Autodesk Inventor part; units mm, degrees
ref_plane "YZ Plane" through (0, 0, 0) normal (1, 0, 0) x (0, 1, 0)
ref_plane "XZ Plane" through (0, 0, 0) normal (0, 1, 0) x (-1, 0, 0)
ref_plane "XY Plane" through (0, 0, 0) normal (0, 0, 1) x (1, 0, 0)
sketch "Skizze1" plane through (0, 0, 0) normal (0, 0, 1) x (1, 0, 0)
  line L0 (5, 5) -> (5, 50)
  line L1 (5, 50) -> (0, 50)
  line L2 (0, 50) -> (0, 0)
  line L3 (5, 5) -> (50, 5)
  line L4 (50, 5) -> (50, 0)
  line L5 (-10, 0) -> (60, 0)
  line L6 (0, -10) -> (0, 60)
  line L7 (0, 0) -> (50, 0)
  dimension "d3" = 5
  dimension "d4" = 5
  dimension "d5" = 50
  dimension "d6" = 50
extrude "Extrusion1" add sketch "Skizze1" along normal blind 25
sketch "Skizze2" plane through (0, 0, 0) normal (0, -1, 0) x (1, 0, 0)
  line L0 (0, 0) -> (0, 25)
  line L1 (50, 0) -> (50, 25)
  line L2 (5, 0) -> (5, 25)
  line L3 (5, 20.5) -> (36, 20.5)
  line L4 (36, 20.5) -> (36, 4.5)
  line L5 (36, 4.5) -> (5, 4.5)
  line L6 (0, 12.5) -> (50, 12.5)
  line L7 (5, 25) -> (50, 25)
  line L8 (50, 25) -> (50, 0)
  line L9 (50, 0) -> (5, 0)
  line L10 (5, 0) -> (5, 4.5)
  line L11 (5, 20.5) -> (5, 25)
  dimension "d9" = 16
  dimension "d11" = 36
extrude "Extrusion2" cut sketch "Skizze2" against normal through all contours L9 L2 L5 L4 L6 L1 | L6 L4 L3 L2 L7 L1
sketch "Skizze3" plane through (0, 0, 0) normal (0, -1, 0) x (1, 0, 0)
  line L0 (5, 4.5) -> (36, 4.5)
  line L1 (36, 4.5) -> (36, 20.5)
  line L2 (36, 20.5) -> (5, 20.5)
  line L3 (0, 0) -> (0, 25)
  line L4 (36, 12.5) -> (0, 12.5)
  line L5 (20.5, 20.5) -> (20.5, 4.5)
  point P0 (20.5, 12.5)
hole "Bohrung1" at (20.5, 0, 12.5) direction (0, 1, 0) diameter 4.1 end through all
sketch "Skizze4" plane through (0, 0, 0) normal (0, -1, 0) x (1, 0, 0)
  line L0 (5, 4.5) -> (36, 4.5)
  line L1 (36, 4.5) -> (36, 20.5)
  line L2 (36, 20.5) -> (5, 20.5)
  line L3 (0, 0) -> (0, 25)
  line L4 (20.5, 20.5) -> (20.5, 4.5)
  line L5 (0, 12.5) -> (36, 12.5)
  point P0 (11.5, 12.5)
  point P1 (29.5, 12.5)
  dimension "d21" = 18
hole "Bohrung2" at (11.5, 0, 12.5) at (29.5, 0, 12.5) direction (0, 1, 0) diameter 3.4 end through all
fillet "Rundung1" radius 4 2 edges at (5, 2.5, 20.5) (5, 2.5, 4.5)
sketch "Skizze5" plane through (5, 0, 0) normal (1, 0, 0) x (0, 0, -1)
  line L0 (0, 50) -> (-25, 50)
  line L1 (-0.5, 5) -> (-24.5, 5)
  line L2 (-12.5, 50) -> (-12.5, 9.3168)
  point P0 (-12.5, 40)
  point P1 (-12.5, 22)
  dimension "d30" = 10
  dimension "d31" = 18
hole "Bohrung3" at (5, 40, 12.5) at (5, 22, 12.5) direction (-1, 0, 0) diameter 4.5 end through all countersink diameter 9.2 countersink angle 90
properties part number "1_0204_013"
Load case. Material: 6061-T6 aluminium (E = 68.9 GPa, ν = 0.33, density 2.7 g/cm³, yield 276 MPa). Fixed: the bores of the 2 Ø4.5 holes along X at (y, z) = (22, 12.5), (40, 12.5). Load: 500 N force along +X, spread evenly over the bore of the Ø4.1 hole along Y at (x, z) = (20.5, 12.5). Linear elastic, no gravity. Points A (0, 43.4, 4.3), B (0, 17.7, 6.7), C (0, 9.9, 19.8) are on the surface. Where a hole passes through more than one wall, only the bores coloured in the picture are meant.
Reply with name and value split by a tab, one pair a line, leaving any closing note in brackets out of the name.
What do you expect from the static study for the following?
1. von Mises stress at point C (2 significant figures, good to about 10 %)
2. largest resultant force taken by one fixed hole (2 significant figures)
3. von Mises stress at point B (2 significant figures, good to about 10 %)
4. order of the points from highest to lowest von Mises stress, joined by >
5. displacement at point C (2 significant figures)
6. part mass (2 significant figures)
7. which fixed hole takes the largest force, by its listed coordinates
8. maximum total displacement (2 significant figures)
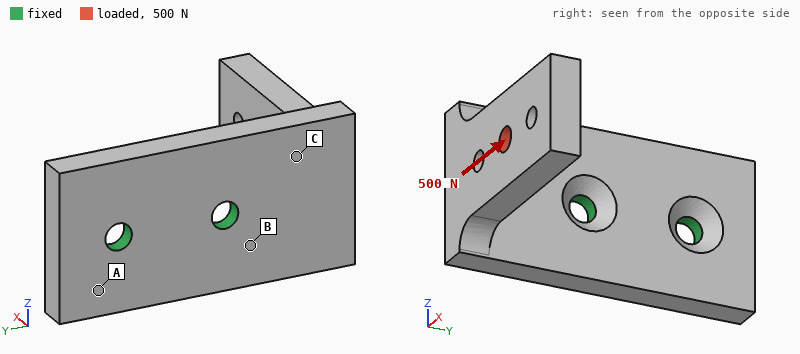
von Mises stress at point C	33 MPa
largest resultant force taken by one fixed hole	920 N
von Mises stress at point B	67 MPa
order of the points from highest to lowest von Mises stress, joined by >	B > C > A
displacement at point C	0.056 mm
part mass	23 g
which fixed hole takes the largest force, by its listed coordinates	(22, 12.5)
maximum total displacement	0.27 mm
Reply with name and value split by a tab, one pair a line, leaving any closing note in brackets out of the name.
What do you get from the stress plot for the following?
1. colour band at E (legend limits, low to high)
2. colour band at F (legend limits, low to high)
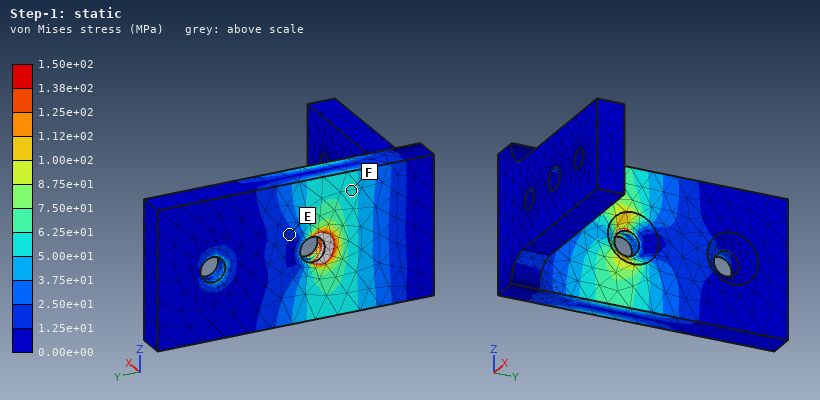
colour band at E	1.25e+01 to 2.50e+01 MPa
colour band at F	5.00e+01 to 6.25e+01 MPa
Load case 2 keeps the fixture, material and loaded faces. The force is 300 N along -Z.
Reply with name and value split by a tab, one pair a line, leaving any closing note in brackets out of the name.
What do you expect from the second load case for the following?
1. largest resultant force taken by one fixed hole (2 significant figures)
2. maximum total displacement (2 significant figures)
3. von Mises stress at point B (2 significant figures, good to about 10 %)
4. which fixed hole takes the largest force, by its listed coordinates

largest resultant force taken by one fixed hole	510 N
maximum total displacement	0.20 mm
von Mises stress at point B	30 MPa
which fixed hole takes the largest force, by its listed coordinates	(22, 12.5)
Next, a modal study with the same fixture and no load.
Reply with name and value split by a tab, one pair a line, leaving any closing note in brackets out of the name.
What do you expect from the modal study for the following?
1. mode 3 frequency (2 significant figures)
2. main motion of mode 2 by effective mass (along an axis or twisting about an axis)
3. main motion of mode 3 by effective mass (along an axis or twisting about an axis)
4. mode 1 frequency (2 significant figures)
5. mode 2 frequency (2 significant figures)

mode 3 frequency	5500 Hz
main motion of mode 2 by effective mass	along Z
main motion of mode 3 by effective mass	along X
mode 1 frequency	2100 Hz
mode 2 frequency	2800 Hz
